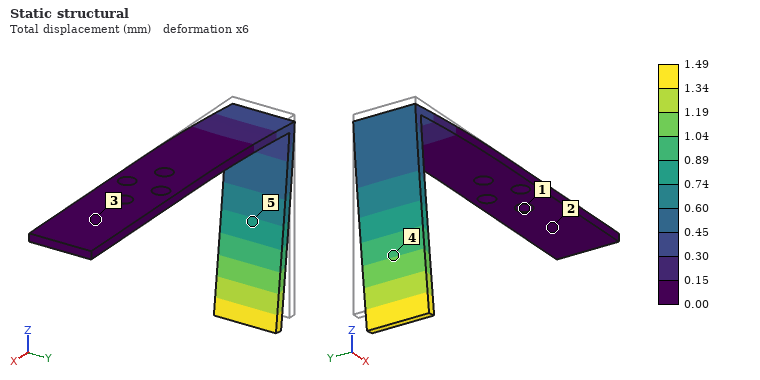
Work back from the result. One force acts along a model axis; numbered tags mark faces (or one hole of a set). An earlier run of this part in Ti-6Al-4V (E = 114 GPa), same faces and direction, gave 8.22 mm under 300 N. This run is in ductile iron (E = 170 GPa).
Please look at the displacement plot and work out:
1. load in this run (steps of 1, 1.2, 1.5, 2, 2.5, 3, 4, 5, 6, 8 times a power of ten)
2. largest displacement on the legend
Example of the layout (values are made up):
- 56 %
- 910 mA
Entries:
- 80 N
- 1.49 mm
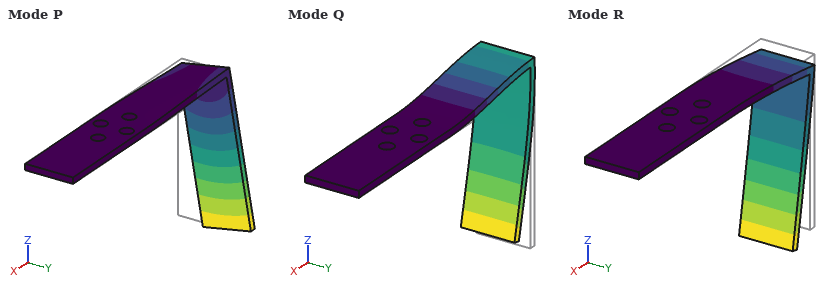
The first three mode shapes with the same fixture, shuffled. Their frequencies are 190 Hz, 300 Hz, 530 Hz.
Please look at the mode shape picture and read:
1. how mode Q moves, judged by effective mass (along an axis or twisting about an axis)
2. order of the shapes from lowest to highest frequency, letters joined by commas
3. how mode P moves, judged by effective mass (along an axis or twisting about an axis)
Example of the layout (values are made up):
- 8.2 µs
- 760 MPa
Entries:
- along Z
- R, P, Q
- along Y
